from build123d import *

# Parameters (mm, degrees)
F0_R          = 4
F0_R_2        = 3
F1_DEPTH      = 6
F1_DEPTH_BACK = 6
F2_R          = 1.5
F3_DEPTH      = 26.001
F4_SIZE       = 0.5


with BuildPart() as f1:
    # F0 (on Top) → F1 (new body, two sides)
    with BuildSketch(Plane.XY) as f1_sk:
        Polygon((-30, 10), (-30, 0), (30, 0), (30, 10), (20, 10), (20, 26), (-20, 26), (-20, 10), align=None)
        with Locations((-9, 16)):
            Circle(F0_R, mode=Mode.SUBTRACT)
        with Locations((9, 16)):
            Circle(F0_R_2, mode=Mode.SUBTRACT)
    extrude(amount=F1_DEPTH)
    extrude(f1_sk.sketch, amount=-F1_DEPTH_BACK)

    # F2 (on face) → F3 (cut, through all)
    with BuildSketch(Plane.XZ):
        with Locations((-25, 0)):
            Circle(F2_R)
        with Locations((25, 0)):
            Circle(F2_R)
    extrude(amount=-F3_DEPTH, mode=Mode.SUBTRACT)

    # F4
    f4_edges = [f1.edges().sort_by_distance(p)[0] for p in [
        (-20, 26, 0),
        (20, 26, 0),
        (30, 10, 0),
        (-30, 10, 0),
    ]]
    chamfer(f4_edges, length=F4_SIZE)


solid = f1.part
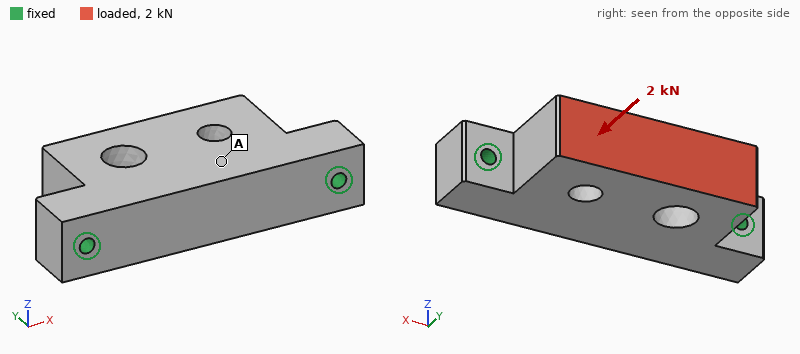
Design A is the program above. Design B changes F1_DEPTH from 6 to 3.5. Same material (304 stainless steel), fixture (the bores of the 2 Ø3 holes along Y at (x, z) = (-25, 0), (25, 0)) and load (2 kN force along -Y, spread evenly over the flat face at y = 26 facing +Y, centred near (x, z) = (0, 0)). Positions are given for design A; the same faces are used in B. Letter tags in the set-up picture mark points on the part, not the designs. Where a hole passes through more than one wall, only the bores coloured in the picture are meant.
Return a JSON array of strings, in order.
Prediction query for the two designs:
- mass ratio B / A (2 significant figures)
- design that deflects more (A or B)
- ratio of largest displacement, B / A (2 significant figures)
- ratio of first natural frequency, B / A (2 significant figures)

["0.79", "B", "1.3", "0.92"]
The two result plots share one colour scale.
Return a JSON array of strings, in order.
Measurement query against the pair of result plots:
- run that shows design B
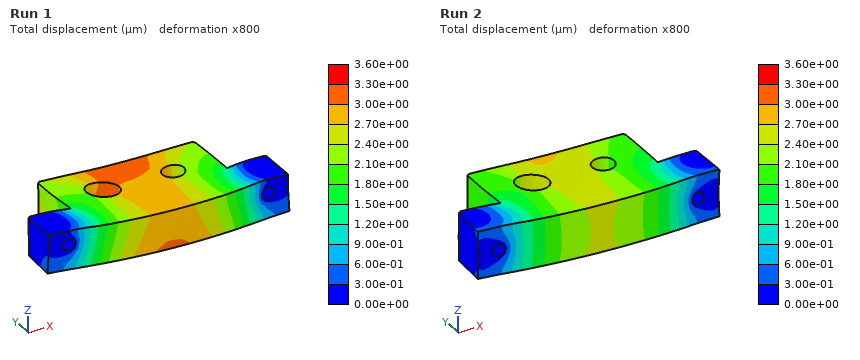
["Run 1"]
